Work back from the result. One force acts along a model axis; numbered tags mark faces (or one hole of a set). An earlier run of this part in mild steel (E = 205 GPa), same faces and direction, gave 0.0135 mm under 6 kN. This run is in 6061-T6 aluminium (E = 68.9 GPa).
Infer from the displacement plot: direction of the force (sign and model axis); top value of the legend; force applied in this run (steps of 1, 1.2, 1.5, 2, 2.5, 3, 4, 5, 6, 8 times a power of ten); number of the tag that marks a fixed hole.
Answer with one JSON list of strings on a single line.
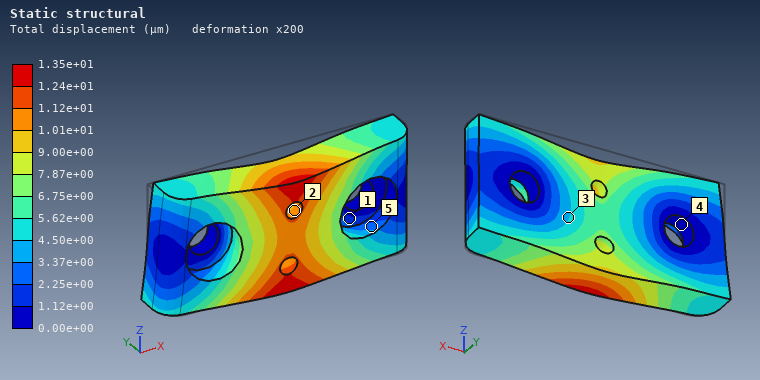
["-Z", "1.35e+01 µm", "2 kN", "4"]
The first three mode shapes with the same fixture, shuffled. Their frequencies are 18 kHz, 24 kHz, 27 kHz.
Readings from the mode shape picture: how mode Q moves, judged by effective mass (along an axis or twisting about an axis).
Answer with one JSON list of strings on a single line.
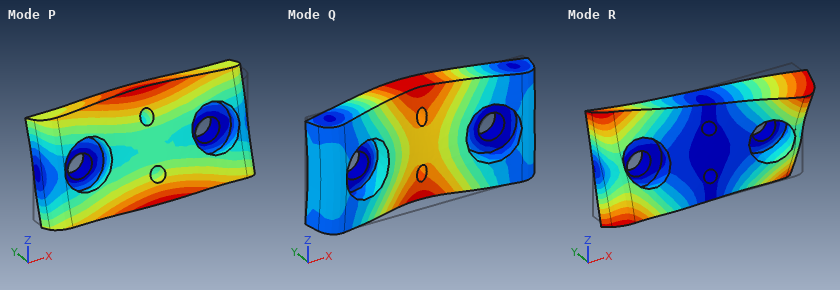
["along Y"]
